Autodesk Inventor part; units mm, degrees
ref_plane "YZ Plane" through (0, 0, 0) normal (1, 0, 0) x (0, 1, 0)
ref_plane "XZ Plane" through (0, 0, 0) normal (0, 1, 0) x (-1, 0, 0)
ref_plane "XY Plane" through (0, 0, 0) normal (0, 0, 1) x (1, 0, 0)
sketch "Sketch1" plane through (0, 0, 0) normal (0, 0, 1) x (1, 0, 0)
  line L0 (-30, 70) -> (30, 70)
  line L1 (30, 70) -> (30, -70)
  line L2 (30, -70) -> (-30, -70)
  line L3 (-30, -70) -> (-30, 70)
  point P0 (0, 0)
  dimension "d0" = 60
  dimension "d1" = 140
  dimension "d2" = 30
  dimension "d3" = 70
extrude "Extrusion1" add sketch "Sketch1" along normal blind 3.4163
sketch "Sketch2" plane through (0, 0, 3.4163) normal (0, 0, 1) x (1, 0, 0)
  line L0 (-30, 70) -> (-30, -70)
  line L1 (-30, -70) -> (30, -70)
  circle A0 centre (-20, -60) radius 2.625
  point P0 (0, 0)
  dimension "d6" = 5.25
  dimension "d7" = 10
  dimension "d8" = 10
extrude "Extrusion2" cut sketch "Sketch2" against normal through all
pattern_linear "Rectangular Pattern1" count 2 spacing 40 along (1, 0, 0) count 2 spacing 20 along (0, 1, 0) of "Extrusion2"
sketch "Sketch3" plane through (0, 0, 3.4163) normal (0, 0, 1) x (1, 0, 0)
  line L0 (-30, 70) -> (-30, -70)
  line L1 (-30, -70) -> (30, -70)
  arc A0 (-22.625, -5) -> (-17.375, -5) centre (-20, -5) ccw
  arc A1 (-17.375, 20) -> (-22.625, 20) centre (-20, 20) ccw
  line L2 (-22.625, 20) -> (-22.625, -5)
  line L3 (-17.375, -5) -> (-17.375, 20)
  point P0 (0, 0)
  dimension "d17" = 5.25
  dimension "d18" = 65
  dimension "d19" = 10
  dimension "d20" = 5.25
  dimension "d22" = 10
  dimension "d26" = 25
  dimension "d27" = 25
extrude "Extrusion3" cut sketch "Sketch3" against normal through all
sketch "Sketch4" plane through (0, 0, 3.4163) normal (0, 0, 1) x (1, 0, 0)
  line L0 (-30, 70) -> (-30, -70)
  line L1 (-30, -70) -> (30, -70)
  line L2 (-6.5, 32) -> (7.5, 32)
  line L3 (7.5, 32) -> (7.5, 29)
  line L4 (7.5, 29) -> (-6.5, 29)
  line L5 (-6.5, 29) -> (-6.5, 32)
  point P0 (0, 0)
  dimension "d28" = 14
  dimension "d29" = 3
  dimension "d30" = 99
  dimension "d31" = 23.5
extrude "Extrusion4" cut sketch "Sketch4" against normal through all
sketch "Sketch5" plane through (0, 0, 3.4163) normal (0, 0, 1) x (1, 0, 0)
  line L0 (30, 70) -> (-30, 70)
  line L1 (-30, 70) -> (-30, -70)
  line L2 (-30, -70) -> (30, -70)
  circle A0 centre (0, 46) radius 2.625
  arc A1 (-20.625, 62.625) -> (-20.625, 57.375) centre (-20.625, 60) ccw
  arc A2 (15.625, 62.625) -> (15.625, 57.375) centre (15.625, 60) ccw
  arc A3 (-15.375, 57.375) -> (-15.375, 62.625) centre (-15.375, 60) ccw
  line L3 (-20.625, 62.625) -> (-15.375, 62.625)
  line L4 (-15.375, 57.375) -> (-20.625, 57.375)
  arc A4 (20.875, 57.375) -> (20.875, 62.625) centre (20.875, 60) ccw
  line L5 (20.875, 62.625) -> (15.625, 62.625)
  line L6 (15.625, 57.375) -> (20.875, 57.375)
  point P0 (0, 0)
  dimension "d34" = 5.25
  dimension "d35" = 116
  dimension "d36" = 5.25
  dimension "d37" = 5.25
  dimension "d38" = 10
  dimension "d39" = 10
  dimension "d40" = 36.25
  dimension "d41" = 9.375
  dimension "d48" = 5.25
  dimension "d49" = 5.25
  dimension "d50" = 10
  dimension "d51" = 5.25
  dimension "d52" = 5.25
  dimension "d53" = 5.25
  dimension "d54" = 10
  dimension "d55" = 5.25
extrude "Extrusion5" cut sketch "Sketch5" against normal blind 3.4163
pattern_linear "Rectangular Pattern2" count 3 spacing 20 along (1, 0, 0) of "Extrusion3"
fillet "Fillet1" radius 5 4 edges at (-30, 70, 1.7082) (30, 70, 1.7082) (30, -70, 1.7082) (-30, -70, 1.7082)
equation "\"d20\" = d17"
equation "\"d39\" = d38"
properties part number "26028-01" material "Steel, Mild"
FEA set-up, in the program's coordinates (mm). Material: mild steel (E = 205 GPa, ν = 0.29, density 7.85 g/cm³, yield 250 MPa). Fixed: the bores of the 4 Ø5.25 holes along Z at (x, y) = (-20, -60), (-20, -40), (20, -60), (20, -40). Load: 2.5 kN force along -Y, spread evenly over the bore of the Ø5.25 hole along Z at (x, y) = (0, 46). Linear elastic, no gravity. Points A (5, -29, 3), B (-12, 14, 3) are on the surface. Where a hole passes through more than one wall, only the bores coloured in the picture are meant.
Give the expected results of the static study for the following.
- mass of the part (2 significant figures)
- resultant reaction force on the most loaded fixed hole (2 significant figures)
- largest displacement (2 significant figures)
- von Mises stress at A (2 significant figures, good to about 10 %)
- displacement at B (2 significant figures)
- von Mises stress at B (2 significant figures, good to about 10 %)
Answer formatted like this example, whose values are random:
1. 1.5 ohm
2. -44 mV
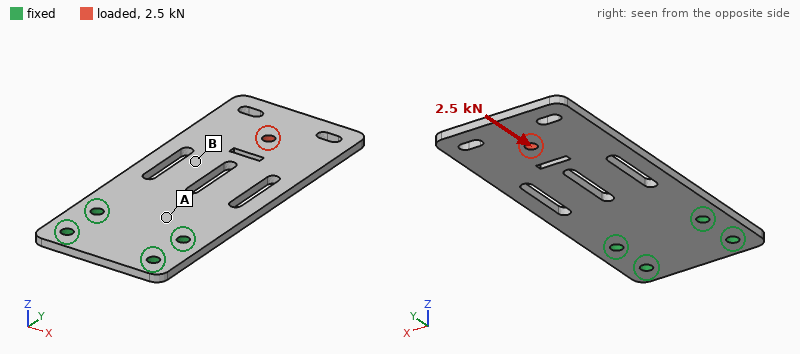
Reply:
1. 210 g
2. 1000 N
3. 9.3 µm
4. 8.6 MPa
5. 4.2 µm
6. 18 MPa
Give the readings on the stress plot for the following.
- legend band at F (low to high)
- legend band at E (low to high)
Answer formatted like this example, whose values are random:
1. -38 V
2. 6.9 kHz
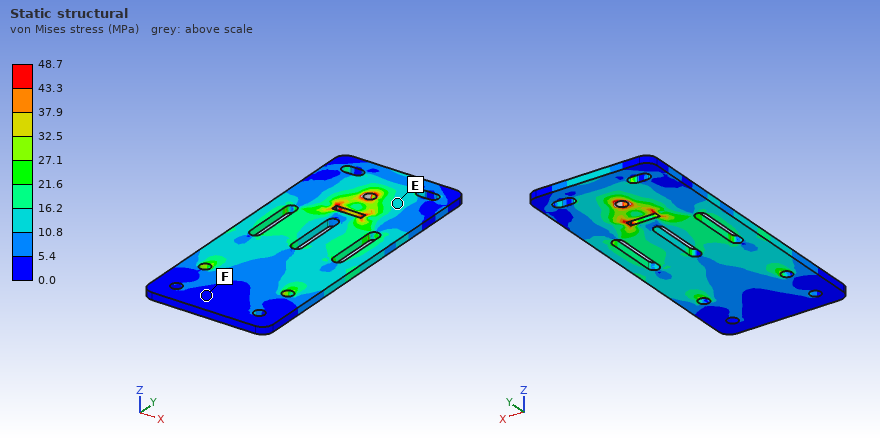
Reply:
1. 0.0 to 5.4 MPa
2. 10.8 to 16.2 MPa
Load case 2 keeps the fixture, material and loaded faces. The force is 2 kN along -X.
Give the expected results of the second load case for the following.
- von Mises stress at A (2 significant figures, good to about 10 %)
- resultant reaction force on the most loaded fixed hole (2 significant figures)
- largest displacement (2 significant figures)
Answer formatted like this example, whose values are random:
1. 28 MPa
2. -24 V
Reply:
1. 25 MPa
2. 3.6 kN
3. 92 µm
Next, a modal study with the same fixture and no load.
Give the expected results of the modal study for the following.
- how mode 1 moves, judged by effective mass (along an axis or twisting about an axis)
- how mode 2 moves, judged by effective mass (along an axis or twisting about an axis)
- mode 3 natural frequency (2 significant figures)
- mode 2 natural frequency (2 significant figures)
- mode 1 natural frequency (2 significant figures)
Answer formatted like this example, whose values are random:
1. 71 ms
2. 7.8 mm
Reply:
1. along Z
2. twisting about Y
3. 1500 Hz
4. 900 Hz
5. 240 Hz
